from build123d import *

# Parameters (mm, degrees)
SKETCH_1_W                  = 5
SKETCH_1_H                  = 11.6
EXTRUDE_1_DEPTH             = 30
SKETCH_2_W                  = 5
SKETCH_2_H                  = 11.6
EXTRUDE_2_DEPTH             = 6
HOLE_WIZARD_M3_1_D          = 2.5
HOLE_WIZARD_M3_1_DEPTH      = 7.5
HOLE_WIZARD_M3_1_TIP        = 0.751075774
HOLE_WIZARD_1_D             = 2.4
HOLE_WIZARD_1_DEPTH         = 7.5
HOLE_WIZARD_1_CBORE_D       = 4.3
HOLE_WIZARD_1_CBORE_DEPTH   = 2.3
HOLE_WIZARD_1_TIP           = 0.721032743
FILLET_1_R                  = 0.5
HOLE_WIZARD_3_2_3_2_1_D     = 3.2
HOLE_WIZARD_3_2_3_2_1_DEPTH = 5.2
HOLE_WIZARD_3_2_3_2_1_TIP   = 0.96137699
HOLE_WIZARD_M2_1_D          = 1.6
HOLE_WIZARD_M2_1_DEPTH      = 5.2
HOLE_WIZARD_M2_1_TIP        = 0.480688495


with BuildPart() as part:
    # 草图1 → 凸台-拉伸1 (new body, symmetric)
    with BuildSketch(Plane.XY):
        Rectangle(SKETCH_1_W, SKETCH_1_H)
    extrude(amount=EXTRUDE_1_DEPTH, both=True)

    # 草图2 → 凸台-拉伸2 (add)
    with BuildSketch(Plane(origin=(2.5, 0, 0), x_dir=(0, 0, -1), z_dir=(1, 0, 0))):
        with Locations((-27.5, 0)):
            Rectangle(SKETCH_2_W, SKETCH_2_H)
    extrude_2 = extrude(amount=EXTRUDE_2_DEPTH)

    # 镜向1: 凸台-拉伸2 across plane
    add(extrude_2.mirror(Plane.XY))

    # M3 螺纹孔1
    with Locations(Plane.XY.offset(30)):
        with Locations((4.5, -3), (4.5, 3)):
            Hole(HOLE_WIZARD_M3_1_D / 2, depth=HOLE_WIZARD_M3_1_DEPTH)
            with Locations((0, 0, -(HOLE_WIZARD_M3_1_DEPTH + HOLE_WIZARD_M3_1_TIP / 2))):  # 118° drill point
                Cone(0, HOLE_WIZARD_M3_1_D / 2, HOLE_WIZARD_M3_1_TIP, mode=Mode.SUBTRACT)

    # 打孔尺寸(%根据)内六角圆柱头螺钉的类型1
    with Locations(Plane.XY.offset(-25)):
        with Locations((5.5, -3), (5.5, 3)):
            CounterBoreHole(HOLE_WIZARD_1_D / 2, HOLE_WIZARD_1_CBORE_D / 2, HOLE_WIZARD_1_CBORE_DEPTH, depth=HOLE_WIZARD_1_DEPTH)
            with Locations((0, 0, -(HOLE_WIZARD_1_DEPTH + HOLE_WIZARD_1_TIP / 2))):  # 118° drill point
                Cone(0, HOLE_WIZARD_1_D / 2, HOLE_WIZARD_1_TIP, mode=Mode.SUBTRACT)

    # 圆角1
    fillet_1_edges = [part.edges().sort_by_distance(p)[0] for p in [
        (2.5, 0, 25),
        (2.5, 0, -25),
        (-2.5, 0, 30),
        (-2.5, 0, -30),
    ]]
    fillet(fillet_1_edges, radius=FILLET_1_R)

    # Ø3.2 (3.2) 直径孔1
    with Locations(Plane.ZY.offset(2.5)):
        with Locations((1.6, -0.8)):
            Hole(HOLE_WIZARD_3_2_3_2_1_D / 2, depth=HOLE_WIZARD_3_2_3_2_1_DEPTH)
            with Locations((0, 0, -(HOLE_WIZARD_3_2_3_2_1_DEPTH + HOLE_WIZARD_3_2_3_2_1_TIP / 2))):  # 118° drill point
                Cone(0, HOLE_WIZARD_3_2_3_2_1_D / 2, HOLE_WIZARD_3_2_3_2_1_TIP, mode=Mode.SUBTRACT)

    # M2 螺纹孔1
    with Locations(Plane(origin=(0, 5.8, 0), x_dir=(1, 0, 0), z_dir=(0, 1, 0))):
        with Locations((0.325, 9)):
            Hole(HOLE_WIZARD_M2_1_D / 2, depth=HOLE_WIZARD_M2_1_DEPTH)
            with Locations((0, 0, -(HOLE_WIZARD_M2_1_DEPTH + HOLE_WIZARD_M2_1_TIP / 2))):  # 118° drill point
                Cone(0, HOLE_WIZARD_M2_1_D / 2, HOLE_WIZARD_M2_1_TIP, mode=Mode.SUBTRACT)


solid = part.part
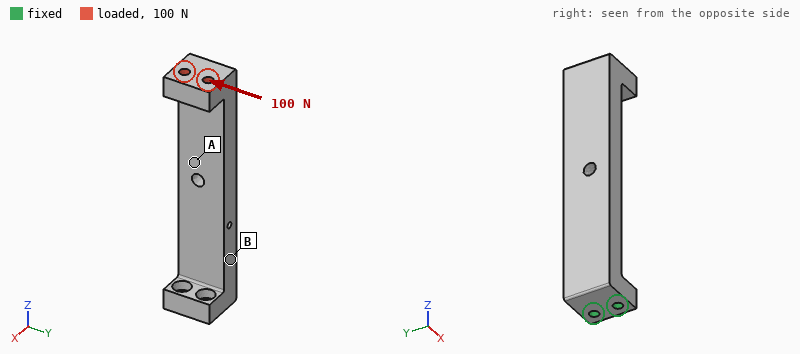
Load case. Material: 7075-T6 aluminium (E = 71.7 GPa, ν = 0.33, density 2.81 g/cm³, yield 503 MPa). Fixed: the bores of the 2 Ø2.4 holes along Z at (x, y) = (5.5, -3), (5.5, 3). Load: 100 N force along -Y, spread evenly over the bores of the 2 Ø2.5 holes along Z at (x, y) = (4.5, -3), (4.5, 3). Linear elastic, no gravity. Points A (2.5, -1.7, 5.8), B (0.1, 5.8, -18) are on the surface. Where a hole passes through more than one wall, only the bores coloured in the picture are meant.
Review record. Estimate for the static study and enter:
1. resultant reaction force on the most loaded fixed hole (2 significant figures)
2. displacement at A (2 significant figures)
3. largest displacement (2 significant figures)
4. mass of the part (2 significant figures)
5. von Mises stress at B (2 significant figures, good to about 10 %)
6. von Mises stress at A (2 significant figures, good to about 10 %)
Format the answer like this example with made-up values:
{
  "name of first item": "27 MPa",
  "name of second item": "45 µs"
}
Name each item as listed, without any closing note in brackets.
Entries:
{
  "resultant reaction force on the most loaded fixed hole": "690 N",
  "displacement at A": "0.13 mm",
  "largest displacement": "0.29 mm",
  "mass of the part": "11 g",
  "von Mises stress at B": "41 MPa",
  "von Mises stress at A": "20 MPa"
}
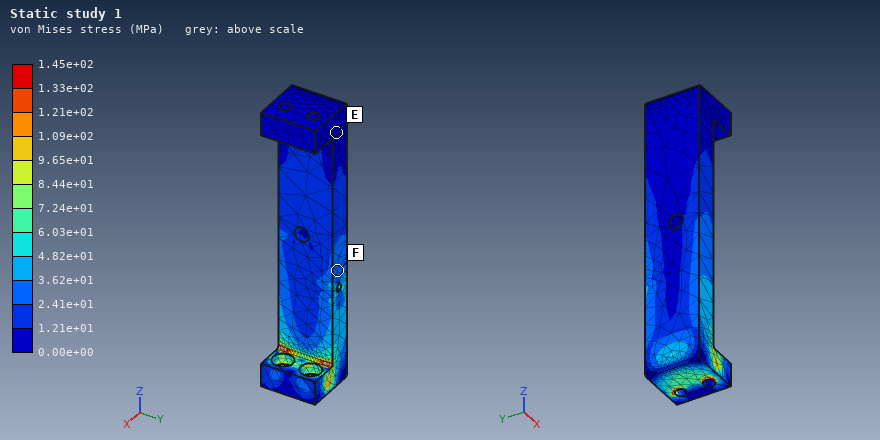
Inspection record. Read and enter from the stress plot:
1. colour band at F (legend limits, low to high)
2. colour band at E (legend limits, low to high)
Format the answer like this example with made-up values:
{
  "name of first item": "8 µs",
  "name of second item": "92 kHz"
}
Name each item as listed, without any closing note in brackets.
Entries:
{
  "colour band at F": "2.41e+01 to 3.62e+01 MPa",
  "colour band at E": "0.00e+00 to 1.21e+01 MPa"
}
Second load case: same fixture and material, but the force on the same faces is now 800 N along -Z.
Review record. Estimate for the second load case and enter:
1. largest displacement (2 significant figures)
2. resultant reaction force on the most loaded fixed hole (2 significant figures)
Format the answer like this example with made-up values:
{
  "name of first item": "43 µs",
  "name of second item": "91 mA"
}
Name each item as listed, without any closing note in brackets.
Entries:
{
  "largest displacement": "0.74 mm",
  "resultant reaction force on the most loaded fixed hole": "400 N"
}
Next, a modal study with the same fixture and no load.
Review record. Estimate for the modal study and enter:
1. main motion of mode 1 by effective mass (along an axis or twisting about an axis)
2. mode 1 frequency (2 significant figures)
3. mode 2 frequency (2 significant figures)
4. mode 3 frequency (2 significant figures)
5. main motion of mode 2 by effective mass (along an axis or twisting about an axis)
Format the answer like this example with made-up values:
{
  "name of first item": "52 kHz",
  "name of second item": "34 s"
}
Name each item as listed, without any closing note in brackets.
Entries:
{
  "main motion of mode 1 by effective mass": "along X",
  "mode 1 frequency": "850 Hz",
  "mode 2 frequency": "1600 Hz",
  "mode 3 frequency": "5300 Hz",
  "main motion of mode 2 by effective mass": "along Y"
}
